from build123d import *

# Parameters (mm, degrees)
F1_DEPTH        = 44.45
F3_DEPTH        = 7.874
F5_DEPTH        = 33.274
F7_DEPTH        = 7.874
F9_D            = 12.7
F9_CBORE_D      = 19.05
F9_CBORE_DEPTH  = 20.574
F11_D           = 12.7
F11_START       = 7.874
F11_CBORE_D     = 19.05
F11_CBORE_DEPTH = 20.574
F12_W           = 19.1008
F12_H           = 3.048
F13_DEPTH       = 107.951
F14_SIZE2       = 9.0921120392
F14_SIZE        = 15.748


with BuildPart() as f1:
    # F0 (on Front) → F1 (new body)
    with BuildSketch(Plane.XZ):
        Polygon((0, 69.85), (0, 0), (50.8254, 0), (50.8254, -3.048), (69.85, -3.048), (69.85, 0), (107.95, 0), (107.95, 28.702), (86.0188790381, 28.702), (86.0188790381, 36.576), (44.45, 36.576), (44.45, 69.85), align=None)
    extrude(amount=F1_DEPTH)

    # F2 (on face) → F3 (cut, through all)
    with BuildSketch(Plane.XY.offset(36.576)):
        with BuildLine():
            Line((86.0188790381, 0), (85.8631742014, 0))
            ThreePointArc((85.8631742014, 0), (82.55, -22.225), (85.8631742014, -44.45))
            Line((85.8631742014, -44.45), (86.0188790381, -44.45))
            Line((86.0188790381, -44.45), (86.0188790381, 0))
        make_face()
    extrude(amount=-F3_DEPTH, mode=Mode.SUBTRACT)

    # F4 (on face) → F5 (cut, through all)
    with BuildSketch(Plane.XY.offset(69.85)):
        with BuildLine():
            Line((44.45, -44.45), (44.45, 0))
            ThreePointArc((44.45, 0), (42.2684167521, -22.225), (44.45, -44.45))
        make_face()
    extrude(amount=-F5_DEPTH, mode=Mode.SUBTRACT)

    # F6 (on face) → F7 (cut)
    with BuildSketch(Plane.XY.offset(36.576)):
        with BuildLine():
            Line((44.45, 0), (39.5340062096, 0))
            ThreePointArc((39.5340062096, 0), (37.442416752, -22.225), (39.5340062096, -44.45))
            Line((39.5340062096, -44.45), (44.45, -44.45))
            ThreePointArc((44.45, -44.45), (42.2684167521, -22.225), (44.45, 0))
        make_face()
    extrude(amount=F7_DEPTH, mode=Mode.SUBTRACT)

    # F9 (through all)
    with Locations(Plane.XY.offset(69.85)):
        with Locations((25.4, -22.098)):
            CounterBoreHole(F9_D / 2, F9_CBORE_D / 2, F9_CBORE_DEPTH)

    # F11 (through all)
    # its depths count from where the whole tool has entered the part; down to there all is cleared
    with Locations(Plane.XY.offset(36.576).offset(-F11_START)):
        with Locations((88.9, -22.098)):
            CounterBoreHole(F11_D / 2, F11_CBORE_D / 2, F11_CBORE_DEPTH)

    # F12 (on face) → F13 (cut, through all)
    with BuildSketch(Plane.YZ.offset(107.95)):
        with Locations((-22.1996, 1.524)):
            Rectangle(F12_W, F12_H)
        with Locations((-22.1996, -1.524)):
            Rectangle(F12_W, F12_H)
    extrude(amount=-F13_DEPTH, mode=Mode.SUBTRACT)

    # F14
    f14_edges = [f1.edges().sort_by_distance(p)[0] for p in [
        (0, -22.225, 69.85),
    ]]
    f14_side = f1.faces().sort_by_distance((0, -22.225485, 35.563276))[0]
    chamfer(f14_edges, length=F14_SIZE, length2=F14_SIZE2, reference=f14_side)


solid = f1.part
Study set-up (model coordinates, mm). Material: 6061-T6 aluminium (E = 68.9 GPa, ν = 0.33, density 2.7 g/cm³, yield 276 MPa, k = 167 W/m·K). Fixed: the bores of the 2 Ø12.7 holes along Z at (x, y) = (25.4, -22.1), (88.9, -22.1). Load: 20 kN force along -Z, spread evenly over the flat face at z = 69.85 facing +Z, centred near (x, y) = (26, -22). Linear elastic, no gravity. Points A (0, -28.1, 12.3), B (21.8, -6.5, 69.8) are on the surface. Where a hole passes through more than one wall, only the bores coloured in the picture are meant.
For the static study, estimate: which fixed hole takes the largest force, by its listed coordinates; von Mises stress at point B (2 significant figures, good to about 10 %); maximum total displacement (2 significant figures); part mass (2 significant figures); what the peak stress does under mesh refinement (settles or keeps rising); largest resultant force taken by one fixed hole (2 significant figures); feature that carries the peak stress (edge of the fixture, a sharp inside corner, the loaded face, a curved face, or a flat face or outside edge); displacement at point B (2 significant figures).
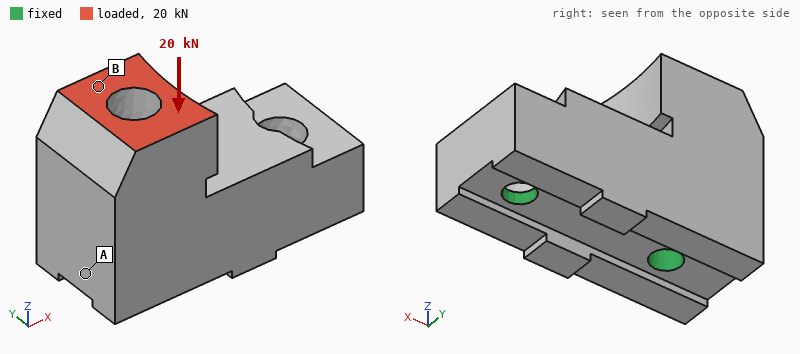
(25.4, -22.1)
16 MPa
16 µm
550 g
keeps rising
20 kN
edge of the fixture
11 µm
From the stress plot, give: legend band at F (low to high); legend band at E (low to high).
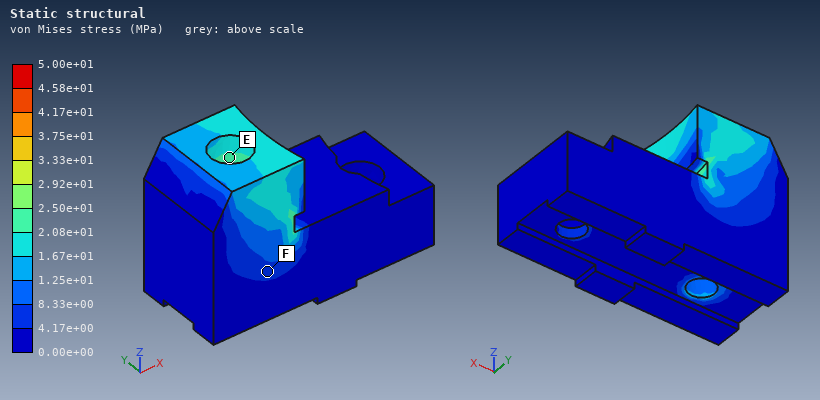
4.17e+00 to 8.33e+00 MPa
2.08e+01 to 2.50e+01 MPa
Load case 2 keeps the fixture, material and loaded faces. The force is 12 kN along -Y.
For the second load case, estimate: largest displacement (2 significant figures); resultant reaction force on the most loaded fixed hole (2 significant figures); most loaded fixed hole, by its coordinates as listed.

42 µm
12 kN
(25.4, -22.1)
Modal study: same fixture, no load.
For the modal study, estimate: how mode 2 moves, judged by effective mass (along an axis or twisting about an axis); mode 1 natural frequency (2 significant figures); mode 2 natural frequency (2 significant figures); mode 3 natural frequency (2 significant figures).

along Z
8500 Hz
12 kHz
13 kHz
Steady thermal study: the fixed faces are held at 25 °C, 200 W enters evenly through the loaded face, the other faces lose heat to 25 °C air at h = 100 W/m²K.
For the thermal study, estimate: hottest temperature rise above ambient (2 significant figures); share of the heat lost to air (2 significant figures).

30 K
6.5 %
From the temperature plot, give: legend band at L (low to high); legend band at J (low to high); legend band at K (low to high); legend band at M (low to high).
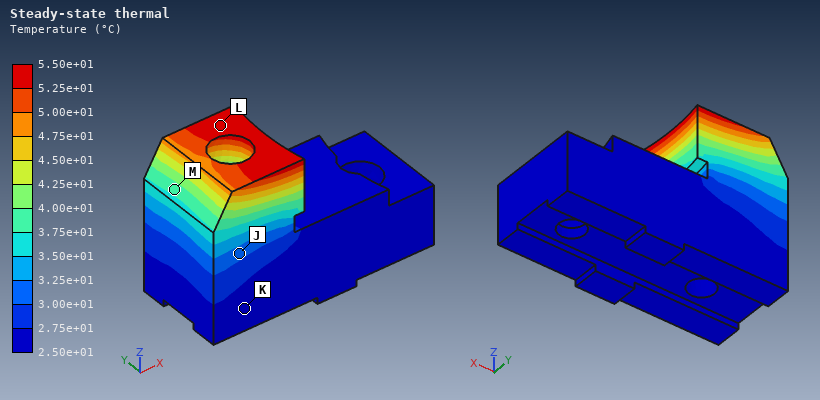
5.25e+01 to 5.50e+01 °C
3.00e+01 to 3.25e+01 °C
2.50e+01 to 2.75e+01 °C
3.75e+01 to 4.00e+01 °C
